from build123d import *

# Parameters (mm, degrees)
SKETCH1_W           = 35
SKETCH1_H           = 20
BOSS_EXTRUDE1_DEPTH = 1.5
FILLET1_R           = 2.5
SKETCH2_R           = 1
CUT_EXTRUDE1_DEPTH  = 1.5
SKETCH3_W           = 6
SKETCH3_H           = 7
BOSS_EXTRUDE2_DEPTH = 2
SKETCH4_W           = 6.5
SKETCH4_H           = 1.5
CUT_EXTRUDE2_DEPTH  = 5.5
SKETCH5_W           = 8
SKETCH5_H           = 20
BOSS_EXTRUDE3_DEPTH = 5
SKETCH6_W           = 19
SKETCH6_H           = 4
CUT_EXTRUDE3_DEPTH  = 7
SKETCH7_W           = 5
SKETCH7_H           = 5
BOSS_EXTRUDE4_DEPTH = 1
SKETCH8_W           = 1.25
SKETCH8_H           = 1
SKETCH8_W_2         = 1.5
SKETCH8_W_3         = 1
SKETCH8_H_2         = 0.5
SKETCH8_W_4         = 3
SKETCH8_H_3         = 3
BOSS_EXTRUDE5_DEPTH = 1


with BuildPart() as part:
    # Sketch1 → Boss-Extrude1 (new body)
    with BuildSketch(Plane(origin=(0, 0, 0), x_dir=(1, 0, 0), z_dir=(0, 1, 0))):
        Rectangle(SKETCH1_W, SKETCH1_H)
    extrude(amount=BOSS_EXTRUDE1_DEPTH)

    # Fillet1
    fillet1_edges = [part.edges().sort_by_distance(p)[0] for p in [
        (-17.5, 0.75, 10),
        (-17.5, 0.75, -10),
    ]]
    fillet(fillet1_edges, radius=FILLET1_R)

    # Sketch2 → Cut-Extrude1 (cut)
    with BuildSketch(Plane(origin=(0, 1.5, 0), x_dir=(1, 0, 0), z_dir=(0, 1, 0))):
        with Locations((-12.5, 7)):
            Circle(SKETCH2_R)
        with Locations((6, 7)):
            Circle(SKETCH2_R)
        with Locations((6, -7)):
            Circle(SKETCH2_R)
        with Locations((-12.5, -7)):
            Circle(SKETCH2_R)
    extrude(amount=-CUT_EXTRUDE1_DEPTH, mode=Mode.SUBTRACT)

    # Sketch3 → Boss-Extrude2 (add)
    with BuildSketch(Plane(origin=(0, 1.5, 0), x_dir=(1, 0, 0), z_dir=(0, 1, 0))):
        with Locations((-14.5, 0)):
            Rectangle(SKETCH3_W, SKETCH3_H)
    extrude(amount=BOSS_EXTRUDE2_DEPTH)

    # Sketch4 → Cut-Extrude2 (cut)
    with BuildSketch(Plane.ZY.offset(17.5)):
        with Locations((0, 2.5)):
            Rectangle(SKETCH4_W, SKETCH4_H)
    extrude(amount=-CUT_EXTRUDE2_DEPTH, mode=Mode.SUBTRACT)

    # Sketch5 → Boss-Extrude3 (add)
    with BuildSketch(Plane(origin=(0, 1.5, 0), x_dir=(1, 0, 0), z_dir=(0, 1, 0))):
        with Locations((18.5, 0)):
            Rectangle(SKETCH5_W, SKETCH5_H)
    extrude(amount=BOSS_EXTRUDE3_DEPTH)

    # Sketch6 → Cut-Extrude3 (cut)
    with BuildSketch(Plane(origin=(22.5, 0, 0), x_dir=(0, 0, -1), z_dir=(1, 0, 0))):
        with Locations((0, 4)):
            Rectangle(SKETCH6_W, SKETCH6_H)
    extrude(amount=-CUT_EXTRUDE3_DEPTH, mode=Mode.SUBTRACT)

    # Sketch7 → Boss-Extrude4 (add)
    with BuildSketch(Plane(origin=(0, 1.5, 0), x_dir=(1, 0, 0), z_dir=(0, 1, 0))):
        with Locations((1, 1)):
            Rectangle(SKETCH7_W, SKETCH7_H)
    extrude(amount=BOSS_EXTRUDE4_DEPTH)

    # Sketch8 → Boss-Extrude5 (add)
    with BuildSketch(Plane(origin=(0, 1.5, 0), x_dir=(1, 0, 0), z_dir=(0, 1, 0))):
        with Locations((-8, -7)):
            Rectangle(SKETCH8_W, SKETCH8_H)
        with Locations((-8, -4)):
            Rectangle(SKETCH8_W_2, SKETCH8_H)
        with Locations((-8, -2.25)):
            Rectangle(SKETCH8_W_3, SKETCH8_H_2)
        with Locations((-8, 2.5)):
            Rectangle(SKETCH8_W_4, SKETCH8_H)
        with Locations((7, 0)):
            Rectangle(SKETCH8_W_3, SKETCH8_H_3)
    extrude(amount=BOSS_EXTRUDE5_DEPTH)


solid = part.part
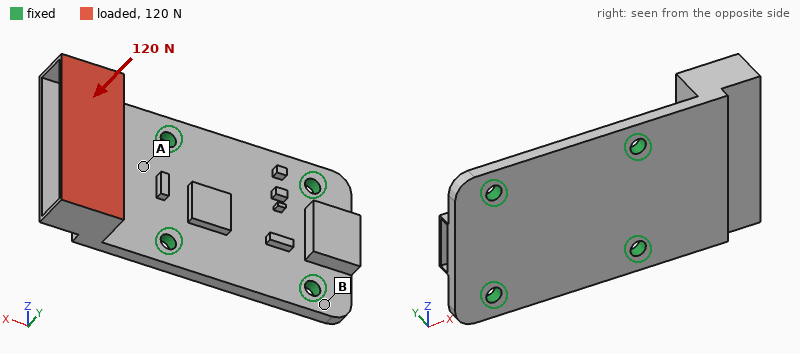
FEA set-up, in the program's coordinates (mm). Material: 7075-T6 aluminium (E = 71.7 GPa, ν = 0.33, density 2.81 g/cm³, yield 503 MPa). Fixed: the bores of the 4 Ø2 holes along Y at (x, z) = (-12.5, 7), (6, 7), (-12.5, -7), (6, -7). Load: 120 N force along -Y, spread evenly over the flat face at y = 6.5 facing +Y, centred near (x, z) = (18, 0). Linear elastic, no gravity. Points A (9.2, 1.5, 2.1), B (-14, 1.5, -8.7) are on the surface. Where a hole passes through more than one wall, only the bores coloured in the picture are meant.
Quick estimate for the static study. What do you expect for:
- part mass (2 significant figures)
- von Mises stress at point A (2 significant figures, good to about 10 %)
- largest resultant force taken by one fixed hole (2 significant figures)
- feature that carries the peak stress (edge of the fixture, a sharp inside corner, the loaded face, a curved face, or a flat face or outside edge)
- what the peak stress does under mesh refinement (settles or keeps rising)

3.8 g
110 MPa
67 N
edge of the fixture
keeps rising
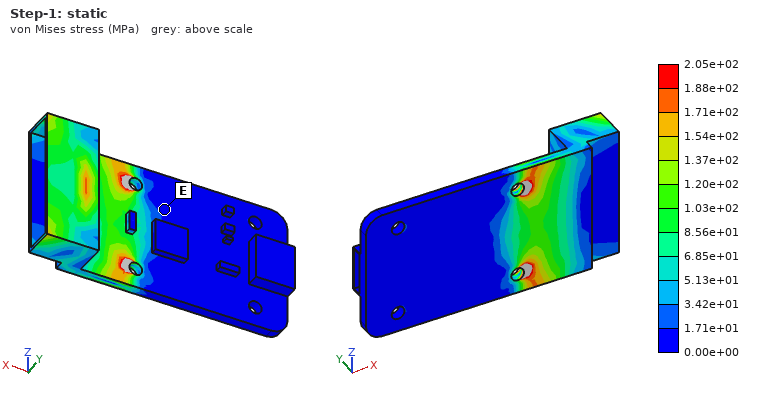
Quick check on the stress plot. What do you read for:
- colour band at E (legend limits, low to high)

0.00e+00 to 1.71e+01 MPa
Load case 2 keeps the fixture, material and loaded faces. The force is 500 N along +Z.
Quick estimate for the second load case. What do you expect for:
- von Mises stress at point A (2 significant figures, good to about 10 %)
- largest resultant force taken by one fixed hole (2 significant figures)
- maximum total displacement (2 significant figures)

130 MPa
500 N
0.13 mm
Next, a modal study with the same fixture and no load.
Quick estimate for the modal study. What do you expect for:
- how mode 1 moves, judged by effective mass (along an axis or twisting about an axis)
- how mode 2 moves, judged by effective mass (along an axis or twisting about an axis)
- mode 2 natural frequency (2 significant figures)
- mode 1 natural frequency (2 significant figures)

along Y
twisting about X
8100 Hz
4100 Hz
